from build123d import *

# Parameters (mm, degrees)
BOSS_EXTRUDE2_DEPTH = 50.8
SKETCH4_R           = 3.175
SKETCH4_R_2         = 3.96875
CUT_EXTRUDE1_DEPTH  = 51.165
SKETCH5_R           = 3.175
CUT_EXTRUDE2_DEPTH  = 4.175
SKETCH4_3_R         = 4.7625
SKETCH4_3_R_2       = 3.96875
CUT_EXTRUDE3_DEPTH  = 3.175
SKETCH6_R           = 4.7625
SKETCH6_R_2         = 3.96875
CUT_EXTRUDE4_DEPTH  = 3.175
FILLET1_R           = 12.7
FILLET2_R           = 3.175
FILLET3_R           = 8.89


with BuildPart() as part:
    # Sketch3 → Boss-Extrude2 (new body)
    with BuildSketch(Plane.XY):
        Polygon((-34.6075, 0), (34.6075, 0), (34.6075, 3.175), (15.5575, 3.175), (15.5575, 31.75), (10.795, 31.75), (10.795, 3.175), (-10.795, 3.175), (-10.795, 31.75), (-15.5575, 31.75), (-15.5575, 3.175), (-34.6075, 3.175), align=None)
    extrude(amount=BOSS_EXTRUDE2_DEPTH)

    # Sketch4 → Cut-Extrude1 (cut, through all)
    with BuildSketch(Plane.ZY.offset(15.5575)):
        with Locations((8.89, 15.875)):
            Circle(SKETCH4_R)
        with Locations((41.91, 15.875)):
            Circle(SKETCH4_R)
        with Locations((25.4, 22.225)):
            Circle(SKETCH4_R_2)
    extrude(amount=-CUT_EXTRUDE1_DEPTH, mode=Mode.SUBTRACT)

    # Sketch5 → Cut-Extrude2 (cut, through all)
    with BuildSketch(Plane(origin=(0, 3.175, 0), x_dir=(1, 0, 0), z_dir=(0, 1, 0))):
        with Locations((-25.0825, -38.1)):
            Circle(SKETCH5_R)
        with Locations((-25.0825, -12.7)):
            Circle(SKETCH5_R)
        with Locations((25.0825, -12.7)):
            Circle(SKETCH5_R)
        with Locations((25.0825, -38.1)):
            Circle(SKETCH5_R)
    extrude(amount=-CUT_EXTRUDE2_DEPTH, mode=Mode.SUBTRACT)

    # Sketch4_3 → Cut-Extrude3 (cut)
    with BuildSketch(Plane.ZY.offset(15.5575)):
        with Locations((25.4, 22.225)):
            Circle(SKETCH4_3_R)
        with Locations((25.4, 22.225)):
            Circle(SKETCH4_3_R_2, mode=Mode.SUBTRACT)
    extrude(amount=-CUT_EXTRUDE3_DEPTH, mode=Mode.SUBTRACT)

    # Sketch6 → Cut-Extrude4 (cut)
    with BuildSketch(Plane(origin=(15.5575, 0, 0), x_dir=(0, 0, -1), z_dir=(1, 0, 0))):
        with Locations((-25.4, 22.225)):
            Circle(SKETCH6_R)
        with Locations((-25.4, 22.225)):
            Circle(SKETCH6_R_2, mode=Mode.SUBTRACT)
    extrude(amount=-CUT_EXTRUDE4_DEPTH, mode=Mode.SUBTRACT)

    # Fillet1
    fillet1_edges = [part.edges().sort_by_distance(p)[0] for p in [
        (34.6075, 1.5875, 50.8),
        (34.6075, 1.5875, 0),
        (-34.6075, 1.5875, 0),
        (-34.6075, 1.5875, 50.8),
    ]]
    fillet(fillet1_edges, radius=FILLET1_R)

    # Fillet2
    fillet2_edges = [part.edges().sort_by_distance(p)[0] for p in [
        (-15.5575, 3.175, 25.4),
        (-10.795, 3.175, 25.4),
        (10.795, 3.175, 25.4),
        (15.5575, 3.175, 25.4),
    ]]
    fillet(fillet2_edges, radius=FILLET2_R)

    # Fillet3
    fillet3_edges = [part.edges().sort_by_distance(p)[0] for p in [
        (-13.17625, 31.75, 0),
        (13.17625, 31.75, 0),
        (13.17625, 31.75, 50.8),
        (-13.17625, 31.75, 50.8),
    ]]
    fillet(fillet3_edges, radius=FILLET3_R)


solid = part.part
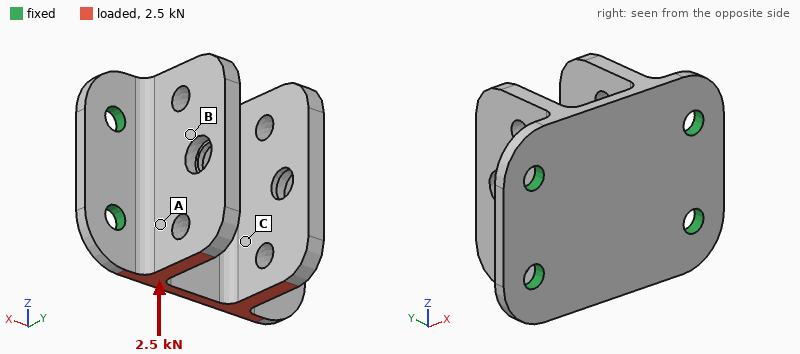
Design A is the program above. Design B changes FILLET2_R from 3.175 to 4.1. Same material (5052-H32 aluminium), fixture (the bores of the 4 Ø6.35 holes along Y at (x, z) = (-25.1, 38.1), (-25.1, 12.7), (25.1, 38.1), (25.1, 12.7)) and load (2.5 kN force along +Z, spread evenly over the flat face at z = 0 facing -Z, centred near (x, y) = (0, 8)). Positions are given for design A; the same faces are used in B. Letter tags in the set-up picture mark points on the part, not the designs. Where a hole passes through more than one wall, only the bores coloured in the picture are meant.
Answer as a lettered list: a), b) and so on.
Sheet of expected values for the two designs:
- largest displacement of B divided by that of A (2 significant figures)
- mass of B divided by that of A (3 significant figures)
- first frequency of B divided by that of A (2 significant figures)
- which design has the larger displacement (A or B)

a) 0.91
b) 1.01
c) 1.0
d) A
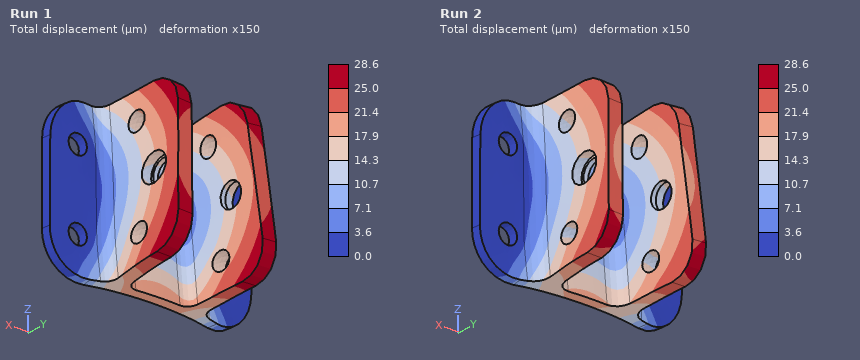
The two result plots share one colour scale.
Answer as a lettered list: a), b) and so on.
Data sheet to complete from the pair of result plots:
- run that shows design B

a) Run 2
